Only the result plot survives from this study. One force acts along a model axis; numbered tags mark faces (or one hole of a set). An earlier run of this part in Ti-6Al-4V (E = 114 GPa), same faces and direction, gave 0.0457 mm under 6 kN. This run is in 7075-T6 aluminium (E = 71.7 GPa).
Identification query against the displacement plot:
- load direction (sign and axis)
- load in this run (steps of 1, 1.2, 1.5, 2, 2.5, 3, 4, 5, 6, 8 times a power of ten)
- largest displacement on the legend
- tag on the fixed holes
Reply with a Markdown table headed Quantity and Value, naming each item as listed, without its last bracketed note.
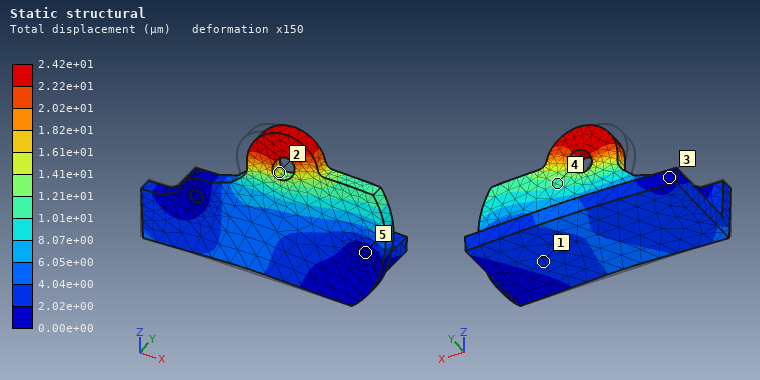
| Quantity | Value |
|---|---|
| load direction | +X |
| load in this run | 2 kN |
| largest displacement on the legend | 2.42e+01 µm |
| tag on the fixed holes | 5 |
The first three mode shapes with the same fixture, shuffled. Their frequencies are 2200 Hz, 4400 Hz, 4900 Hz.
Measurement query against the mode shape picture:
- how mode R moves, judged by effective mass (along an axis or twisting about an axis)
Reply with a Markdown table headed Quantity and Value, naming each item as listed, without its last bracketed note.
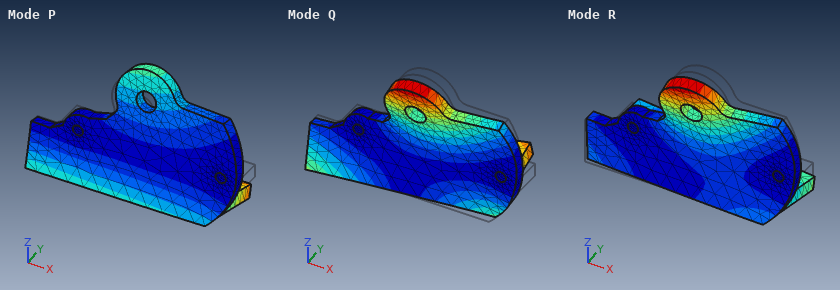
| Quantity | Value |
|---|---|
| how mode R moves, judged by effective mass | along Y |
